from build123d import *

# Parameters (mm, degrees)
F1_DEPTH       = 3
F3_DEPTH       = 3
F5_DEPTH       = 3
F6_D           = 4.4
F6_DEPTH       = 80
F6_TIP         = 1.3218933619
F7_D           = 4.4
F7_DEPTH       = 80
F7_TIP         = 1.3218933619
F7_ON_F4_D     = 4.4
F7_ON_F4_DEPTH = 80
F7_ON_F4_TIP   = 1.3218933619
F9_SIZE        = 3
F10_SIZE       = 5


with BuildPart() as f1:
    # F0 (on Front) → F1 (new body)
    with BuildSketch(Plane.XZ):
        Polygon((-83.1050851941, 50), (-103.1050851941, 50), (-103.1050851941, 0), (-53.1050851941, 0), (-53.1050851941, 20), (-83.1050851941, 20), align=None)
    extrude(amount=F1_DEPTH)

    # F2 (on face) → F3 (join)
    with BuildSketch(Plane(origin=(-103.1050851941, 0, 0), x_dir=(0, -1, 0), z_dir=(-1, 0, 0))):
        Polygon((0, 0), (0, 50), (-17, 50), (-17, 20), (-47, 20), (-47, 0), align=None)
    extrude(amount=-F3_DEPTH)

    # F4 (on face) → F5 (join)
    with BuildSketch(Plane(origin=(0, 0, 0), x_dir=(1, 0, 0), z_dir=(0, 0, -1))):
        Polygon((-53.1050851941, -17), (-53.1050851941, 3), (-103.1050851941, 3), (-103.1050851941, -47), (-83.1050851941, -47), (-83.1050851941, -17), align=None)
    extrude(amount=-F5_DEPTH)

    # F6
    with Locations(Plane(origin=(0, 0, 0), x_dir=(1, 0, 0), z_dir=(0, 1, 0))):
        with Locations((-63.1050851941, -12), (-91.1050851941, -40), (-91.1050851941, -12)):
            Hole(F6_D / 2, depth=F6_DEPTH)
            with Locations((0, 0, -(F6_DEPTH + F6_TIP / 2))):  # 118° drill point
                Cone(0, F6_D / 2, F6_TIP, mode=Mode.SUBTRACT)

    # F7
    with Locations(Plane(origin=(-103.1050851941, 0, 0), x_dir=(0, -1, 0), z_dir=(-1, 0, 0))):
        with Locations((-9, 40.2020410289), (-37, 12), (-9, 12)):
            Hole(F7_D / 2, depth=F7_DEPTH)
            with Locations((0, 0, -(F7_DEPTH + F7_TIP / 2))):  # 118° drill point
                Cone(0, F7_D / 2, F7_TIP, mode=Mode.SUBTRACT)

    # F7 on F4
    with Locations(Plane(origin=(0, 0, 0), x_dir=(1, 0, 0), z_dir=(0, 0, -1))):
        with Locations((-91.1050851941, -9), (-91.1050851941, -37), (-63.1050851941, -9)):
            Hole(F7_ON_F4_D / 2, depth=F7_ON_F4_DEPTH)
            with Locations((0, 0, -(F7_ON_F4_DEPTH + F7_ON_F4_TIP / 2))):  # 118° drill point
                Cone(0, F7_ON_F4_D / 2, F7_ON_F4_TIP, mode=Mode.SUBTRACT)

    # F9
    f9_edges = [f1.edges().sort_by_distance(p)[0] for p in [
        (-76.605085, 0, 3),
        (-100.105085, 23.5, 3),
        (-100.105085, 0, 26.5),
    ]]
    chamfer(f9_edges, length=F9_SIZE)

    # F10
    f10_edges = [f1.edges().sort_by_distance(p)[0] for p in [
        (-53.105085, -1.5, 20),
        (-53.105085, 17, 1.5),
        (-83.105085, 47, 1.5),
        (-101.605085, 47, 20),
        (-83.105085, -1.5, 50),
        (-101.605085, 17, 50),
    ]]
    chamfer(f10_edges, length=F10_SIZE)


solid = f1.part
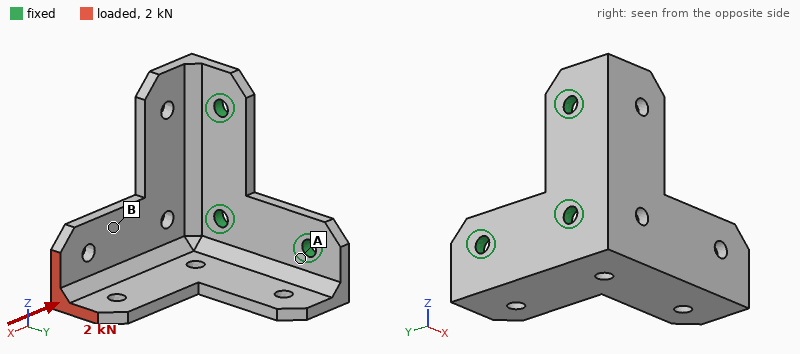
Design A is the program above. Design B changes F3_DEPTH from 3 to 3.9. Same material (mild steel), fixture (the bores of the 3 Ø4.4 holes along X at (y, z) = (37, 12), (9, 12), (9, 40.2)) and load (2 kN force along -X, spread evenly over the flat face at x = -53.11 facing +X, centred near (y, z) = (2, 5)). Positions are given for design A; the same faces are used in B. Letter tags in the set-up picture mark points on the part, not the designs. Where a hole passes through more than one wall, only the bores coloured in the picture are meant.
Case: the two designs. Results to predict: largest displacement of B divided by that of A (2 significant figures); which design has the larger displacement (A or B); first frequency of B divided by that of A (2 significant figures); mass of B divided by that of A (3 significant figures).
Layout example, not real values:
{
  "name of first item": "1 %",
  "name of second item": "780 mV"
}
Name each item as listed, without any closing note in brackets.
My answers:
{
  "largest displacement of B divided by that of A": "0.71",
  "which design has the larger displacement": "A",
  "first frequency of B divided by that of A": "1.2",
  "mass of B divided by that of A": "1.09"
}
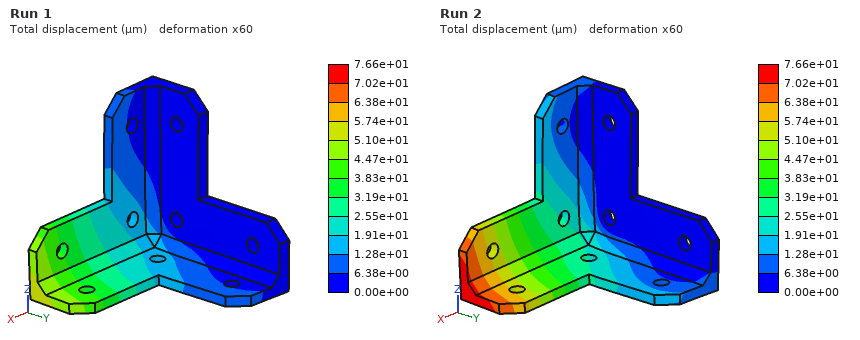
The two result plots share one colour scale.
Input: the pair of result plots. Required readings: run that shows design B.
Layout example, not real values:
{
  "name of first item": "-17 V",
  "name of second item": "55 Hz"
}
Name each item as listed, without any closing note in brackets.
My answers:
{
  "run that shows design B": "Run 1"
}
